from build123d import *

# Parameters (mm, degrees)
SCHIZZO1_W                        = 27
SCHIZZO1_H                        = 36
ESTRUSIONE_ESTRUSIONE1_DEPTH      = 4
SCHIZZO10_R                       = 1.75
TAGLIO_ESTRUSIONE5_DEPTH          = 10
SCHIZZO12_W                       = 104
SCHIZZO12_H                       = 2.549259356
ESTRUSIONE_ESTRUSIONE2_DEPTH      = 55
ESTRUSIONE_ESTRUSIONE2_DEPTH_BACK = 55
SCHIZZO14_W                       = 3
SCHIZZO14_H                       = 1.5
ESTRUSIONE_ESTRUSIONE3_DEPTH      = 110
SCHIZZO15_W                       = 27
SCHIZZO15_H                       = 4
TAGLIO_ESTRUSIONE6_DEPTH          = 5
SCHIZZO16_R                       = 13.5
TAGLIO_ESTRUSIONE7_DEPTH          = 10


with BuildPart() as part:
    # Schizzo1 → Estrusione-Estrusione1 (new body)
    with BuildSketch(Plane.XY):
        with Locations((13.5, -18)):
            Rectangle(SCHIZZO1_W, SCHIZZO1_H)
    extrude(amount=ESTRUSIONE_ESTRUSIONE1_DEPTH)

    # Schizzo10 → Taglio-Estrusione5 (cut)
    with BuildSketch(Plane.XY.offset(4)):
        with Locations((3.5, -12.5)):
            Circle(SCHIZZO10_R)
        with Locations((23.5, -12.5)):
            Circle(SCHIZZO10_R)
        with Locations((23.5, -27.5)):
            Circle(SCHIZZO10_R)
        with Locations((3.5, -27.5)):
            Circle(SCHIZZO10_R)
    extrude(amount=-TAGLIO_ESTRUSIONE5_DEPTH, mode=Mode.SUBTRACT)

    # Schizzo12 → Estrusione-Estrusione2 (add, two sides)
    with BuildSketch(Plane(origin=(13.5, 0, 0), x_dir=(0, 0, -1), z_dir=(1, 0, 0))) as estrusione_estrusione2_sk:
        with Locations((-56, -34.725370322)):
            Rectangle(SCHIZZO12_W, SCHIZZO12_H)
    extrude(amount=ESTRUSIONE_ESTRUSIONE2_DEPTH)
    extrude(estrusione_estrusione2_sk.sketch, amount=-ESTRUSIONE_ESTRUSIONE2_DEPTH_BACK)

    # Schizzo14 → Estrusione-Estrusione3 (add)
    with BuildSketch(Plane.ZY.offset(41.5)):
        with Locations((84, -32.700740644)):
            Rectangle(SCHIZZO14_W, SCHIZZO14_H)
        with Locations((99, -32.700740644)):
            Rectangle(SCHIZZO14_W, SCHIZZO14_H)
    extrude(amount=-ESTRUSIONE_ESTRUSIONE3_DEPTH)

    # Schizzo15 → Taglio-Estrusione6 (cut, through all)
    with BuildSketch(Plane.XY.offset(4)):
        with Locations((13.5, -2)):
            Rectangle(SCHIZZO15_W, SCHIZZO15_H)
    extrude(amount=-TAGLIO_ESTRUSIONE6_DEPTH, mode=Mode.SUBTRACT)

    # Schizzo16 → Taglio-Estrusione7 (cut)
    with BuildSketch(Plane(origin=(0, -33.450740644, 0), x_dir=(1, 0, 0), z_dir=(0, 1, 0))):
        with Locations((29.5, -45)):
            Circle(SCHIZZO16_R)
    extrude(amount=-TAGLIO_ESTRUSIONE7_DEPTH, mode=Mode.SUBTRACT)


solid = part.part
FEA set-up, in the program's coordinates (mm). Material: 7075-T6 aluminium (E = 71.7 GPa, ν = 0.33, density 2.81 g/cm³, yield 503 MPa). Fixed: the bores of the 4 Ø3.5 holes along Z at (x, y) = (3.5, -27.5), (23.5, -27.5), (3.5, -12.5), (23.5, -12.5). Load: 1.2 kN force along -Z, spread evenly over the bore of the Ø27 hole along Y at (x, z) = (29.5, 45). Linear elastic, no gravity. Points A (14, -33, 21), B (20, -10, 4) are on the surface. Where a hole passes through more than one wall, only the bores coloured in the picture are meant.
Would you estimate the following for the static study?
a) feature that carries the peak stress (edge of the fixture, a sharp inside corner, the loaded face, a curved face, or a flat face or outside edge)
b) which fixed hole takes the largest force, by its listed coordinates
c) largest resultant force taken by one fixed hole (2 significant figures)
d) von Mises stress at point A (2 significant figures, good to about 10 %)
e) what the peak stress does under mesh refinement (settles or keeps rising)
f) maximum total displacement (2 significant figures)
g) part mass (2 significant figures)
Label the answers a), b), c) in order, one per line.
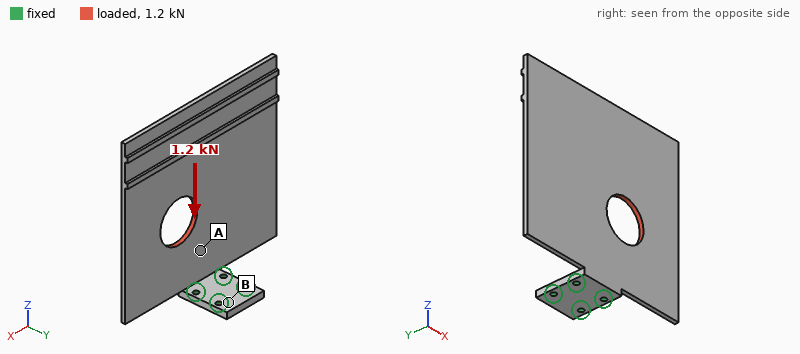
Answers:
a) edge of the fixture
b) (23.5, -27.5)
c) 1.6 kN
d) 23 MPa
e) keeps rising
f) 0.59 mm
g) 90 g
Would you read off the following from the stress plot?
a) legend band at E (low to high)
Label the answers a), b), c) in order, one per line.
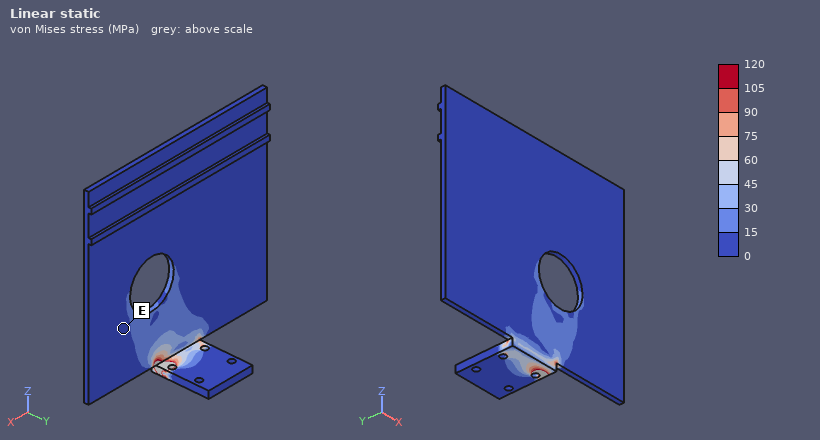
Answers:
a) 0 to 15 MPa
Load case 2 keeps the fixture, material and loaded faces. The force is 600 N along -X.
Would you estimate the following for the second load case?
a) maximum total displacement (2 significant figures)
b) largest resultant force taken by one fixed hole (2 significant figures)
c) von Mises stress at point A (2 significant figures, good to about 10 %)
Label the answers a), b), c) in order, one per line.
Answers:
a) 0.50 mm
b) 1.3 kN
c) 26 MPa
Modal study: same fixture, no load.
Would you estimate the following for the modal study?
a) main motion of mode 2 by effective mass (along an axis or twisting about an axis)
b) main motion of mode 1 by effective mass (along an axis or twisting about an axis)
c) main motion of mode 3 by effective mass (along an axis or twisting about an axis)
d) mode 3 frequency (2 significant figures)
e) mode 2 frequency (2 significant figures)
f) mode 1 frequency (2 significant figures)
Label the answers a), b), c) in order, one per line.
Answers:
a) twisting about Z
b) along Y
c) along X
d) 650 Hz
e) 260 Hz
f) 120 Hz
